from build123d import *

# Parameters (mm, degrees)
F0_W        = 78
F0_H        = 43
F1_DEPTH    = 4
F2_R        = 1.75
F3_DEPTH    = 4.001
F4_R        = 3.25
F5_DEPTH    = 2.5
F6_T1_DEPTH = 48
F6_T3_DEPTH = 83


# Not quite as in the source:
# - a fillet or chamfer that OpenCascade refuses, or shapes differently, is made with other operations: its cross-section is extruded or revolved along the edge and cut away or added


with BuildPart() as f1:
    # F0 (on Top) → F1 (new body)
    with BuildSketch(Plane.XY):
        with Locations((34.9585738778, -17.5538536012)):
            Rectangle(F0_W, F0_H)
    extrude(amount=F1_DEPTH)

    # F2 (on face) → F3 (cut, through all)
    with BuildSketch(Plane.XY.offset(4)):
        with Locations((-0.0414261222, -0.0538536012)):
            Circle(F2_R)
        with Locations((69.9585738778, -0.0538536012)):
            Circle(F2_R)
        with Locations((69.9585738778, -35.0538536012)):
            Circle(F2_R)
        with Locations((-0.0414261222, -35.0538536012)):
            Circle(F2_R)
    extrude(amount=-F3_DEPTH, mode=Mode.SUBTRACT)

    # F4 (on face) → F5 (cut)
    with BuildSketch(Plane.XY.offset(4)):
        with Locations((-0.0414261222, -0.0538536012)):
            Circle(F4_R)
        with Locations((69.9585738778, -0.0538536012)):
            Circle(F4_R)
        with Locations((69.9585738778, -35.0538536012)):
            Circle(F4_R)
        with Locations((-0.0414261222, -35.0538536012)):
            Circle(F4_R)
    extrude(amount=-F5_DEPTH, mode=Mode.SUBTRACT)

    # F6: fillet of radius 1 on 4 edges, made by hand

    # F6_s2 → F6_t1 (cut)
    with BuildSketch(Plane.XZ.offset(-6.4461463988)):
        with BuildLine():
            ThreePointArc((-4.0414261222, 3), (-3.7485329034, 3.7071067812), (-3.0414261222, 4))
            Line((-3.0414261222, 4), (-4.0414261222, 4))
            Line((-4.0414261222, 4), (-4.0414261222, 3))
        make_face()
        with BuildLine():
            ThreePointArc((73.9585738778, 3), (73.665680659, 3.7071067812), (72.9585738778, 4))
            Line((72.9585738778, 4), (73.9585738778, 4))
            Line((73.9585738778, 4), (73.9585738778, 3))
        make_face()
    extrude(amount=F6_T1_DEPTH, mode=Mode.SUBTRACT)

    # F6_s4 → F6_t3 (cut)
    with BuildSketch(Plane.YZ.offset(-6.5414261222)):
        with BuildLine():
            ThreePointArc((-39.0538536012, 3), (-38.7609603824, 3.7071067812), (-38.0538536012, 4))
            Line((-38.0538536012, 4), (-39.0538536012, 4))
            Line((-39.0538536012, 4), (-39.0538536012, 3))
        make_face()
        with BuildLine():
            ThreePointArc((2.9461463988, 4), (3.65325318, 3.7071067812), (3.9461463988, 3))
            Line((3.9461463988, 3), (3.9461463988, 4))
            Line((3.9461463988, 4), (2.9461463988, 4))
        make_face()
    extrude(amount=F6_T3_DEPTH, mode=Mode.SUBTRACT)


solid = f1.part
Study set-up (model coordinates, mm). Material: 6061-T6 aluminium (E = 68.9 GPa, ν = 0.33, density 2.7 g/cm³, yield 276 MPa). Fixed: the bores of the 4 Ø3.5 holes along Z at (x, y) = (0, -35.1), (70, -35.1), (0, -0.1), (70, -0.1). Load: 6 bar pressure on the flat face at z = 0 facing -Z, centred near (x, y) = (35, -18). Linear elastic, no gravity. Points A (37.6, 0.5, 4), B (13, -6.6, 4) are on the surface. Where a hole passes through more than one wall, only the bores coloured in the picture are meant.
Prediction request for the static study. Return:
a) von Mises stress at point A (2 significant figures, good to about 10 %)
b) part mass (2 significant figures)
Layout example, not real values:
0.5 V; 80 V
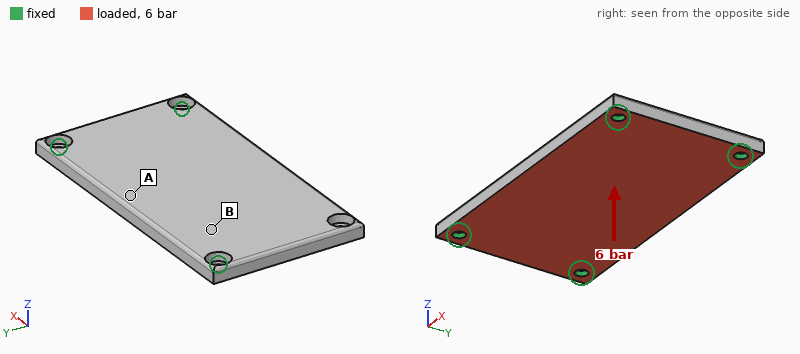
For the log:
82 MPa; 35 g
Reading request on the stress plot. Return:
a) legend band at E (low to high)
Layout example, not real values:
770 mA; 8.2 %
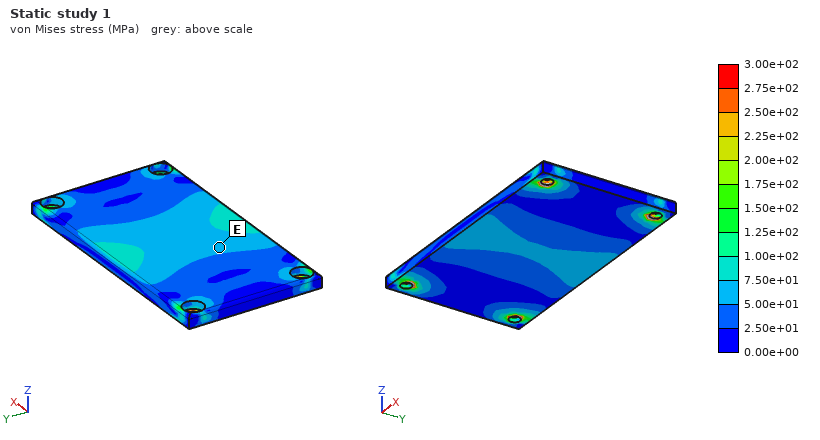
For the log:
5.00e+01 to 7.50e+01 MPa
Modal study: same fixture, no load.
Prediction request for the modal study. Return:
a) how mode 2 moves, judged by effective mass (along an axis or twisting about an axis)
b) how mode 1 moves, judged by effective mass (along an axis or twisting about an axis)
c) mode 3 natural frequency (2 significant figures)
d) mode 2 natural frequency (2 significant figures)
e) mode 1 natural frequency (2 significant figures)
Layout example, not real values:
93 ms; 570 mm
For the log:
twisting about X; along Z; 8200 Hz; 5300 Hz; 2900 Hz
